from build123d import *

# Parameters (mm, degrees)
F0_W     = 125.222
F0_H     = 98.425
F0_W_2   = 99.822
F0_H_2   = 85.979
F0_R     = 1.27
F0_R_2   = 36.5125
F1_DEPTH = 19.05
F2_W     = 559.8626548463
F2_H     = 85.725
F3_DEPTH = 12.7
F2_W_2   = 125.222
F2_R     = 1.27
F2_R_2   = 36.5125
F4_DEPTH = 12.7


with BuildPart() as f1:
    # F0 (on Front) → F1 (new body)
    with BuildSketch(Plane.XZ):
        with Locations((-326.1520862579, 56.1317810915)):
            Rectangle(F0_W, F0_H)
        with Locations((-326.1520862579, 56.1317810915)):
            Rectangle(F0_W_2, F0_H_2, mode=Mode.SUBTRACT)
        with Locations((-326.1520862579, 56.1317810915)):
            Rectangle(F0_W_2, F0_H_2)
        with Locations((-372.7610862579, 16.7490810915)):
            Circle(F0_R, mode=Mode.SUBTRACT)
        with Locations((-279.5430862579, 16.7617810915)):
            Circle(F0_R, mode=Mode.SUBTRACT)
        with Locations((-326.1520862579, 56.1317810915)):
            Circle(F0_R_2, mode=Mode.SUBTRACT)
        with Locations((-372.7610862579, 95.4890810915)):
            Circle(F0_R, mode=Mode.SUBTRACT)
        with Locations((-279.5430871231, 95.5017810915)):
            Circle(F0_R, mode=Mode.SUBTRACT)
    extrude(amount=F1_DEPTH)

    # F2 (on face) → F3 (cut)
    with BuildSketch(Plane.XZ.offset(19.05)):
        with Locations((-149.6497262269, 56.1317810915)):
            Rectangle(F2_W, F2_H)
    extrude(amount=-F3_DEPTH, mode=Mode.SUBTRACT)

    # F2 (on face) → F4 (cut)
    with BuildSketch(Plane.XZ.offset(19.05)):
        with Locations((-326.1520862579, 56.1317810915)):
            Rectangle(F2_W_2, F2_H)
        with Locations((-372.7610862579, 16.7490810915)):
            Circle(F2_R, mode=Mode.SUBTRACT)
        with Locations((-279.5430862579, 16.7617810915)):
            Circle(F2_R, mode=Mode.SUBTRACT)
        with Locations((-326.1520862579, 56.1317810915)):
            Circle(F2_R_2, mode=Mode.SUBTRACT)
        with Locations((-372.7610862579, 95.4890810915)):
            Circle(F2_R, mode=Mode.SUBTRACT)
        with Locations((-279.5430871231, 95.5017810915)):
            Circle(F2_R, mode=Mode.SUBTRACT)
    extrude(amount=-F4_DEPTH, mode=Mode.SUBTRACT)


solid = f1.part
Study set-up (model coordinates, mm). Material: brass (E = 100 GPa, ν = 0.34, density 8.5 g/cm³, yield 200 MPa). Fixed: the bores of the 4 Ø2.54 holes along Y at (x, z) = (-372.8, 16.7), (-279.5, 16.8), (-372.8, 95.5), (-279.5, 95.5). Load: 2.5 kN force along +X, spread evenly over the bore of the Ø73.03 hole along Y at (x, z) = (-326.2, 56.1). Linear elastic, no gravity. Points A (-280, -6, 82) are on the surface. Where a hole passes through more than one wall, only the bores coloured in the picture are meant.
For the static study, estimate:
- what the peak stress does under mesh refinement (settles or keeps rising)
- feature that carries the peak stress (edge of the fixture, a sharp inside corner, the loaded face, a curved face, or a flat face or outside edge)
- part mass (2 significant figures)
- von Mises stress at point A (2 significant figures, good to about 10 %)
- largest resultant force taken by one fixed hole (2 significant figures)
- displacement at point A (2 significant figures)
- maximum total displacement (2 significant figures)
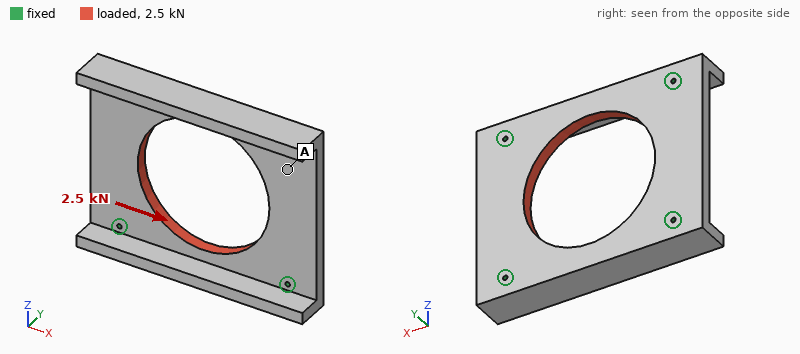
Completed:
keeps rising
edge of the fixture
610 g
2.5 MPa
630 N
1.8 µm
3.4 µm
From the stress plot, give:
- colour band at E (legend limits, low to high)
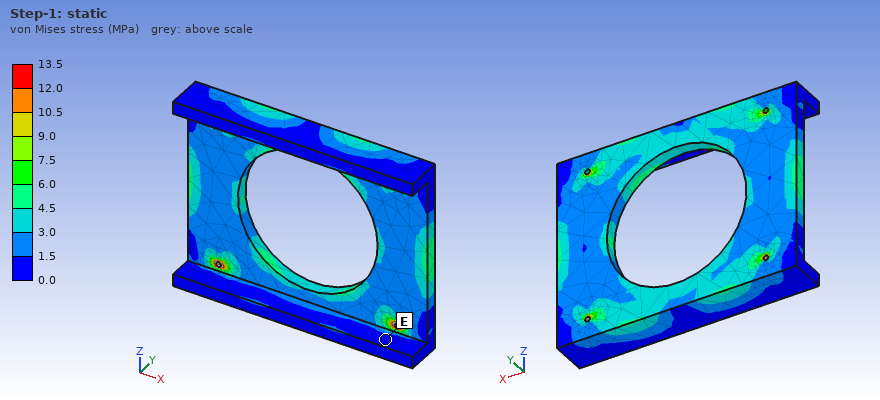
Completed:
0.0 to 1.5 MPa
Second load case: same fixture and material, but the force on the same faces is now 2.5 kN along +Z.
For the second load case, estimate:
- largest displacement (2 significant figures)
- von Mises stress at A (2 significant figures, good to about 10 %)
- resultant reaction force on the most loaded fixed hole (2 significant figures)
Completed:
6.3 µm
4.4 MPa
630 N
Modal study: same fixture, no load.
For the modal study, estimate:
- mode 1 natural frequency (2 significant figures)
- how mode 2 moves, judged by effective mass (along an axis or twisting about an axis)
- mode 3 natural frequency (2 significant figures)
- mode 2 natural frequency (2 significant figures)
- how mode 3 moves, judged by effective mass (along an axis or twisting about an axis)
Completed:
2700 Hz
twisting about Z
3500 Hz
3000 Hz
along Y
